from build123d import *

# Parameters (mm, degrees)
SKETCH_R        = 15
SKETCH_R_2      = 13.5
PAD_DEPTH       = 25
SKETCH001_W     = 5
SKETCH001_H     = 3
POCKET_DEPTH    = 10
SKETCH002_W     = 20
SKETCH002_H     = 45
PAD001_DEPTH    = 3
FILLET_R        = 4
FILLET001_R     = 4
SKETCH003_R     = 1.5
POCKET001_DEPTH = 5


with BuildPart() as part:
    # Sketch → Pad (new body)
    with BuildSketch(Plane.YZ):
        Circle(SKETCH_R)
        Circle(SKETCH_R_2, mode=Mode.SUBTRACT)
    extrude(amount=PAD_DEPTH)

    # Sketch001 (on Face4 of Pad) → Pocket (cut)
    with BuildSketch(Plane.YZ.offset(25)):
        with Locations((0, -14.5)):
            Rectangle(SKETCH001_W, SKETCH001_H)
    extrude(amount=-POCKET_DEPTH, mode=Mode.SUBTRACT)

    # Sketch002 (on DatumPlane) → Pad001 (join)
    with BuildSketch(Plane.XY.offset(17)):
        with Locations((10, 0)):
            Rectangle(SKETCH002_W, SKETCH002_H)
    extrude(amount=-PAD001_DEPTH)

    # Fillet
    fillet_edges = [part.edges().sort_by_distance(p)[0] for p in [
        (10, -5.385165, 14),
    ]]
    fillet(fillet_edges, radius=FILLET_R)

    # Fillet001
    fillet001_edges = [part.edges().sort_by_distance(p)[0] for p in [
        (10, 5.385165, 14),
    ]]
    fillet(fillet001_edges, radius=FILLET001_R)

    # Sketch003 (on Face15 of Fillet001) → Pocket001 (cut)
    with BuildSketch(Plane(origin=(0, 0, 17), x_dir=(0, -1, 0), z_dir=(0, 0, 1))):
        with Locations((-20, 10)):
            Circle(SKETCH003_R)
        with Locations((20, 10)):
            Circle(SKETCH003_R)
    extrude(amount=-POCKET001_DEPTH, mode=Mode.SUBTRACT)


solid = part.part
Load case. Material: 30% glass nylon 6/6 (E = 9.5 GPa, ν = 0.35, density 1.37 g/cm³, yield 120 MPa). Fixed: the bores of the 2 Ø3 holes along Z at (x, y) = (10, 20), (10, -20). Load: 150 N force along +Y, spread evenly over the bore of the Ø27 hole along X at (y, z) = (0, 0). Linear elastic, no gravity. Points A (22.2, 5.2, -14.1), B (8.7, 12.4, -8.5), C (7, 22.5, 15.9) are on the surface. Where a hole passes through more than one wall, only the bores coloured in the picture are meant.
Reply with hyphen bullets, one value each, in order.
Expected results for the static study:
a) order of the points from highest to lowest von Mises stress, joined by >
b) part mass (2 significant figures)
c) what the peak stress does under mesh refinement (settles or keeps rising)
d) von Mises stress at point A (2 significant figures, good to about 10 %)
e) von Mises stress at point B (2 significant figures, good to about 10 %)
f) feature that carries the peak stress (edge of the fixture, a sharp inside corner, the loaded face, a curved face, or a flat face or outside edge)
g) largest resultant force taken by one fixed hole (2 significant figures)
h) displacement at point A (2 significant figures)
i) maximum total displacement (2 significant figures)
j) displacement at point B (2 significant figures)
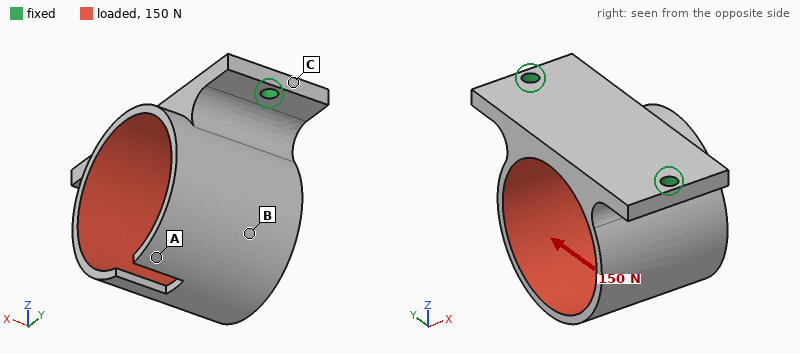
- B > A > C
- 8.9 g
- keeps rising
- 8.6 MPa
- 17 MPa
- a sharp inside corner
- 100 N
- 0.53 mm
- 0.55 mm
- 0.46 mm
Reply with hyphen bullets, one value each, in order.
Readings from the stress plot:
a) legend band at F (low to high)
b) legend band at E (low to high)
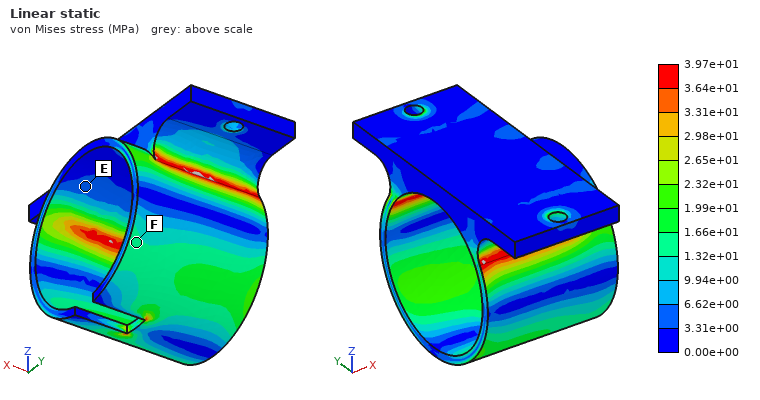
- 1.32e+01 to 1.66e+01 MPa
- 3.31e+00 to 6.62e+00 MPa
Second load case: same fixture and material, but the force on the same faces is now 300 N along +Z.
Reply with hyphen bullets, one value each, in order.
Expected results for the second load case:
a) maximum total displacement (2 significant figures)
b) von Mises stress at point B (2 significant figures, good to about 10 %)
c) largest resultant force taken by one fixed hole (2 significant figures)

- 0.27 mm
- 5.4 MPa
- 170 N
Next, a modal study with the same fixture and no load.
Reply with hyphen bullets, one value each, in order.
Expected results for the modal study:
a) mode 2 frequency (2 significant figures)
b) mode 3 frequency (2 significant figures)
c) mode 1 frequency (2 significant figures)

- 1400 Hz
- 3400 Hz
- 1400 Hz
